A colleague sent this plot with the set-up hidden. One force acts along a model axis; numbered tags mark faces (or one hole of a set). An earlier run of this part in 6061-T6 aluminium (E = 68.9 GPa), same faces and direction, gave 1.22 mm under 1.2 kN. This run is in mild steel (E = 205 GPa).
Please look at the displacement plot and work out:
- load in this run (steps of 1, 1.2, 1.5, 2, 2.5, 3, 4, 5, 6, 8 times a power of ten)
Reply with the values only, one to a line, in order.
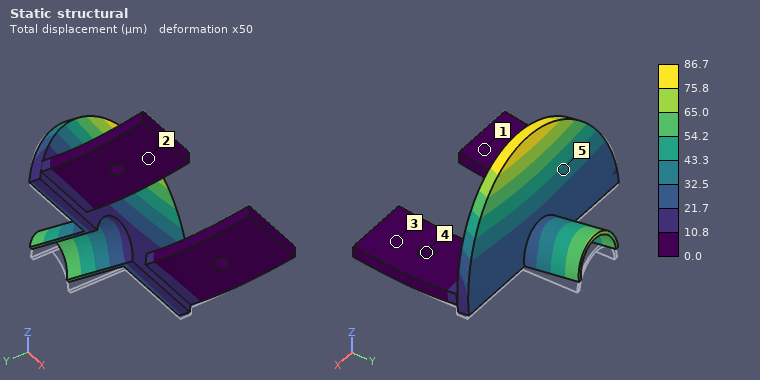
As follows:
250 N
